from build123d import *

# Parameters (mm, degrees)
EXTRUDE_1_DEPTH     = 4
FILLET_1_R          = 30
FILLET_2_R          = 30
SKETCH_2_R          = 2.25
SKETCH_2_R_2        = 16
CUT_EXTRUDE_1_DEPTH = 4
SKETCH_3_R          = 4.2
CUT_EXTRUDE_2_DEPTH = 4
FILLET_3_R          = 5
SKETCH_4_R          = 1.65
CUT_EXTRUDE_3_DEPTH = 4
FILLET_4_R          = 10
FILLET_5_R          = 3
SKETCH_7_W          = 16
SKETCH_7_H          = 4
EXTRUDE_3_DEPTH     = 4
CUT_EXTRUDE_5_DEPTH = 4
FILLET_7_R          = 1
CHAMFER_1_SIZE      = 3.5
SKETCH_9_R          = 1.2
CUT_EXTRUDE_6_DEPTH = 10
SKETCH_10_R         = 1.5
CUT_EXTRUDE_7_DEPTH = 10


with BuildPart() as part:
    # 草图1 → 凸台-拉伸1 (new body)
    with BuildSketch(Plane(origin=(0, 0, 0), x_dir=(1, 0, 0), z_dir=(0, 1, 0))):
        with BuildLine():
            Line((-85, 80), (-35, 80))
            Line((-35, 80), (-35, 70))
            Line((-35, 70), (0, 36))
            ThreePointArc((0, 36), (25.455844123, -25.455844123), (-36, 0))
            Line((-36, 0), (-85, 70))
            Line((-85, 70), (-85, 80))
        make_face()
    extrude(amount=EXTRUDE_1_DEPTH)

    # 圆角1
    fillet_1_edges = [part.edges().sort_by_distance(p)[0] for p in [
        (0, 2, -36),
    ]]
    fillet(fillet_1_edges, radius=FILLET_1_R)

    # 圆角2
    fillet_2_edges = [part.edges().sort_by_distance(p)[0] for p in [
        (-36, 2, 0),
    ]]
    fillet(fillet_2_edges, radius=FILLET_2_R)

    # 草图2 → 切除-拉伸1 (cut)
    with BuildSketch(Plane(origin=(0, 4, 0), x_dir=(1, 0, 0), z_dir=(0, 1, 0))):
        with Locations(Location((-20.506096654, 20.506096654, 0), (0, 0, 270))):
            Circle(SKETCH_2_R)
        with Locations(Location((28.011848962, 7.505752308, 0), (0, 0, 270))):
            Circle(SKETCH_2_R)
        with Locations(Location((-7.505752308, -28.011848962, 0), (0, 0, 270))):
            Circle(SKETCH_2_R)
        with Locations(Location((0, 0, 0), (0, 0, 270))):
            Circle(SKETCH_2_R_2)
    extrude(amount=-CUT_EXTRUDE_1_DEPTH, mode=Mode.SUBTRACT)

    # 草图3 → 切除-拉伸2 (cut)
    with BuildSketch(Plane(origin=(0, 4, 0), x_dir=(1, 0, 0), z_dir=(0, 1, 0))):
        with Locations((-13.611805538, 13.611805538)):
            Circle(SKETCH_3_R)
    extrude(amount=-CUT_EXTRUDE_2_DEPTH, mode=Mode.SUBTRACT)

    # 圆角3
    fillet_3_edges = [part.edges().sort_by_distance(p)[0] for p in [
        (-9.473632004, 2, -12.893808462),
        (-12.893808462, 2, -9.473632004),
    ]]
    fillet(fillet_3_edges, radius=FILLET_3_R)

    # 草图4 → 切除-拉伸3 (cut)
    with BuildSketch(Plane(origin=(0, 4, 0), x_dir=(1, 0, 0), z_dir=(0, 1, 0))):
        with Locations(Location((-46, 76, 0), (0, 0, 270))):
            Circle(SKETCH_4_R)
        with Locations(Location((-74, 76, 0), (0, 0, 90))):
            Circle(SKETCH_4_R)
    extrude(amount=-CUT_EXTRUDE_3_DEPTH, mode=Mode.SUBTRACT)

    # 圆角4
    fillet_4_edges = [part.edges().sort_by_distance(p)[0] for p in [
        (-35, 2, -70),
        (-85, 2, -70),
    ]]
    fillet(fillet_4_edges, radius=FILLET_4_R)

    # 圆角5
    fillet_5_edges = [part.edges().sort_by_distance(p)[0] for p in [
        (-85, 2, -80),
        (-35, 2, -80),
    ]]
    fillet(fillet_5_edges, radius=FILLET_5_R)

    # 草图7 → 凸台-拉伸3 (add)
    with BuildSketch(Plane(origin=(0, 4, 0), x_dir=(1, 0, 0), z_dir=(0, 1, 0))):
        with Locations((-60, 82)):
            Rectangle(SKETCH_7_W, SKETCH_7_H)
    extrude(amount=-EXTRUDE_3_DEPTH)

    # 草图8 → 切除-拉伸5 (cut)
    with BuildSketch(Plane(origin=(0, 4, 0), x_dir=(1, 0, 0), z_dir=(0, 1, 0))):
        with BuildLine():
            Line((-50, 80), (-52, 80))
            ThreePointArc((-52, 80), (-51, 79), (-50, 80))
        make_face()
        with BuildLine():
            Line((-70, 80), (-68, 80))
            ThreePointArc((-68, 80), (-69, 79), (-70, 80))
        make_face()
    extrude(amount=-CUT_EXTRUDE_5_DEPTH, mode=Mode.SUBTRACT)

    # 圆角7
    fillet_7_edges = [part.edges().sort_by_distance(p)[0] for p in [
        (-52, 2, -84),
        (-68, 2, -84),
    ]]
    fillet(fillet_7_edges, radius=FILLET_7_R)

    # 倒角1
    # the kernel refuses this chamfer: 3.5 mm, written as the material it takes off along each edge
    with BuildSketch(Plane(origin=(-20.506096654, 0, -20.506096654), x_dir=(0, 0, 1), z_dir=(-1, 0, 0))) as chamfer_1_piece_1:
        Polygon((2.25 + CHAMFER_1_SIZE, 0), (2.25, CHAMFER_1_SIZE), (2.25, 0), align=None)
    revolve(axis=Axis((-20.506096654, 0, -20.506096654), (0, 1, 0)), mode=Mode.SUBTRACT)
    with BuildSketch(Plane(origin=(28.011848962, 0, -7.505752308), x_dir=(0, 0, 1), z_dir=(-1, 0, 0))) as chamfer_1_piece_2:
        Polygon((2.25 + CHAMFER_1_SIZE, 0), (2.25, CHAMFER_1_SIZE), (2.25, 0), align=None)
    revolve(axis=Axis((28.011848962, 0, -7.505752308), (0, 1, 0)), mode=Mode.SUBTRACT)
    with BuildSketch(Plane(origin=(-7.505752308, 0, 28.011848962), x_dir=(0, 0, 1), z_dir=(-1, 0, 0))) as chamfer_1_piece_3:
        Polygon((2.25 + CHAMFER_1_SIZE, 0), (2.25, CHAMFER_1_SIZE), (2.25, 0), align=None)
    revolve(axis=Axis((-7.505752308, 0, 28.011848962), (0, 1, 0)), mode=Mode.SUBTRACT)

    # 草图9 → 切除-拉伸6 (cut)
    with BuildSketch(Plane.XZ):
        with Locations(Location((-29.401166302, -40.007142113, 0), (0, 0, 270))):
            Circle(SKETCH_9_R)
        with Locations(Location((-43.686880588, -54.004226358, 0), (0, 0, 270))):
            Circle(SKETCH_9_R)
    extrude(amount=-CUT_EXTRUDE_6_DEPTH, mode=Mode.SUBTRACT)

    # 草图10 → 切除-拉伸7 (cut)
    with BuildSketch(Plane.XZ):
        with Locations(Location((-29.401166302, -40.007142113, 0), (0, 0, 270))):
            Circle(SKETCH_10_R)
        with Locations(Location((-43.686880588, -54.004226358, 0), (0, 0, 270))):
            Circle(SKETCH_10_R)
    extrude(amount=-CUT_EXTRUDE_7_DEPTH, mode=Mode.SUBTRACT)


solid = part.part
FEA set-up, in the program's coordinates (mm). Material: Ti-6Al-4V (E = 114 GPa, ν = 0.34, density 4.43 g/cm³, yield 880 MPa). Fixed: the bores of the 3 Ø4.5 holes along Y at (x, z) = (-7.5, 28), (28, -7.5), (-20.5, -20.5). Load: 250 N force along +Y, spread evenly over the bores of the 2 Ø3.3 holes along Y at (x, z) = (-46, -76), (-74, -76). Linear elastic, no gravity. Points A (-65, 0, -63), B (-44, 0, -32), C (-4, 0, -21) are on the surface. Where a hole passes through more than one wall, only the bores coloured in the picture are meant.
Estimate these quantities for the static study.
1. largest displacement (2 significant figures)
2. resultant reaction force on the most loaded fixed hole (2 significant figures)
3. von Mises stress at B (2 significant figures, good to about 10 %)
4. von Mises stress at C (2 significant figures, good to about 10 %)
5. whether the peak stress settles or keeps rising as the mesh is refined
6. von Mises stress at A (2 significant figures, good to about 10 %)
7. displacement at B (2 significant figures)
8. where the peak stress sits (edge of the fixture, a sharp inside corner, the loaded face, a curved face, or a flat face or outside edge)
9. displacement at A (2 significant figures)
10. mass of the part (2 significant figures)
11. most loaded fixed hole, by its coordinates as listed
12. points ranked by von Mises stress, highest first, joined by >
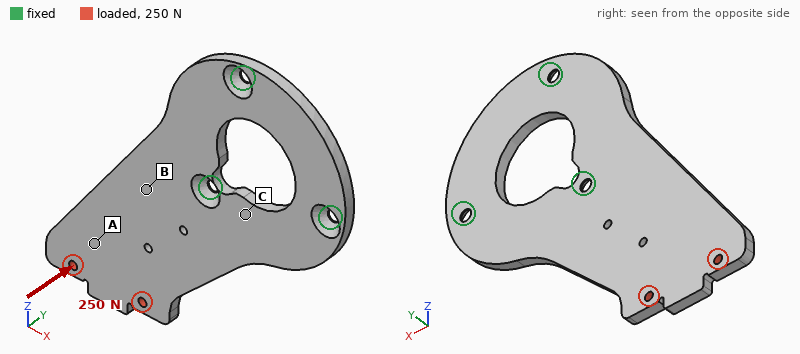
1.7 mm
1.9 kN
89 MPa
58 MPa
keeps rising
26 MPa
0.26 mm
edge of the fixture
1.1 mm
110 g
(-20.5, -20.5)
B > C > A
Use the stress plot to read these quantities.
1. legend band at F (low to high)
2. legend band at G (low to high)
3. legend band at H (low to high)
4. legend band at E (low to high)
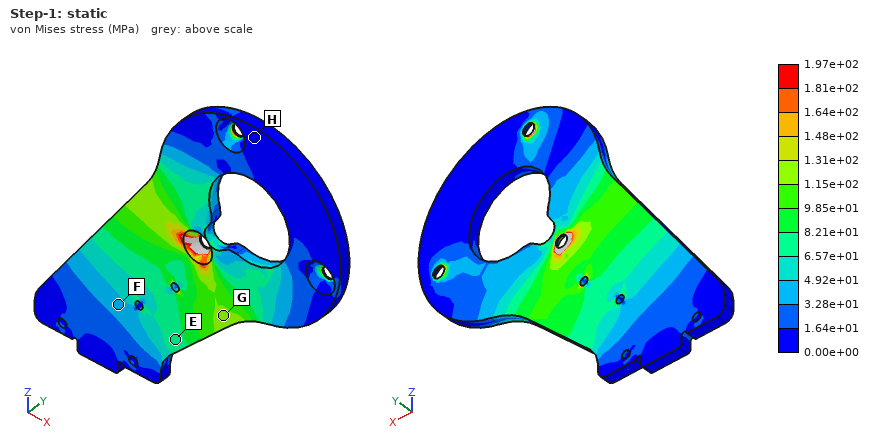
3.28e+01 to 4.92e+01 MPa
1.15e+02 to 1.31e+02 MPa
0.00e+00 to 1.64e+01 MPa
6.57e+01 to 8.21e+01 MPa
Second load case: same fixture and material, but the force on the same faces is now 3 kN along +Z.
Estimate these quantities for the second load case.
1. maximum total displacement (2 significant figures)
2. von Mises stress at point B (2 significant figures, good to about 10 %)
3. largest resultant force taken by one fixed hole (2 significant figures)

0.20 mm
42 MPa
2.7 kN
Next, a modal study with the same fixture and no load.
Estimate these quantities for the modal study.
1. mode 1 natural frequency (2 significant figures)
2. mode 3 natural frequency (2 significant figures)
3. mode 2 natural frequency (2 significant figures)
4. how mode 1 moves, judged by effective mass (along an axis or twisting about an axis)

490 Hz
2600 Hz
1400 Hz
along Y
